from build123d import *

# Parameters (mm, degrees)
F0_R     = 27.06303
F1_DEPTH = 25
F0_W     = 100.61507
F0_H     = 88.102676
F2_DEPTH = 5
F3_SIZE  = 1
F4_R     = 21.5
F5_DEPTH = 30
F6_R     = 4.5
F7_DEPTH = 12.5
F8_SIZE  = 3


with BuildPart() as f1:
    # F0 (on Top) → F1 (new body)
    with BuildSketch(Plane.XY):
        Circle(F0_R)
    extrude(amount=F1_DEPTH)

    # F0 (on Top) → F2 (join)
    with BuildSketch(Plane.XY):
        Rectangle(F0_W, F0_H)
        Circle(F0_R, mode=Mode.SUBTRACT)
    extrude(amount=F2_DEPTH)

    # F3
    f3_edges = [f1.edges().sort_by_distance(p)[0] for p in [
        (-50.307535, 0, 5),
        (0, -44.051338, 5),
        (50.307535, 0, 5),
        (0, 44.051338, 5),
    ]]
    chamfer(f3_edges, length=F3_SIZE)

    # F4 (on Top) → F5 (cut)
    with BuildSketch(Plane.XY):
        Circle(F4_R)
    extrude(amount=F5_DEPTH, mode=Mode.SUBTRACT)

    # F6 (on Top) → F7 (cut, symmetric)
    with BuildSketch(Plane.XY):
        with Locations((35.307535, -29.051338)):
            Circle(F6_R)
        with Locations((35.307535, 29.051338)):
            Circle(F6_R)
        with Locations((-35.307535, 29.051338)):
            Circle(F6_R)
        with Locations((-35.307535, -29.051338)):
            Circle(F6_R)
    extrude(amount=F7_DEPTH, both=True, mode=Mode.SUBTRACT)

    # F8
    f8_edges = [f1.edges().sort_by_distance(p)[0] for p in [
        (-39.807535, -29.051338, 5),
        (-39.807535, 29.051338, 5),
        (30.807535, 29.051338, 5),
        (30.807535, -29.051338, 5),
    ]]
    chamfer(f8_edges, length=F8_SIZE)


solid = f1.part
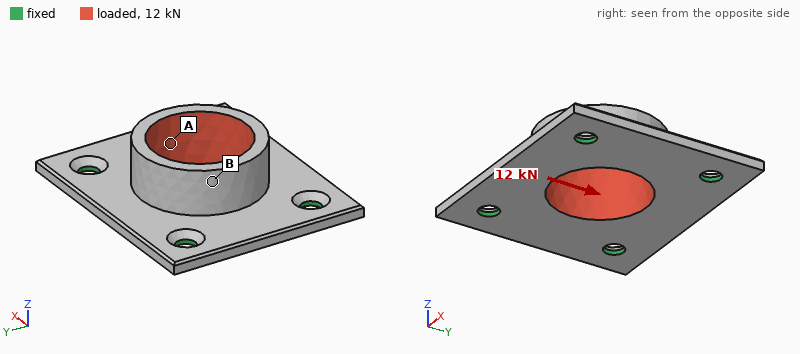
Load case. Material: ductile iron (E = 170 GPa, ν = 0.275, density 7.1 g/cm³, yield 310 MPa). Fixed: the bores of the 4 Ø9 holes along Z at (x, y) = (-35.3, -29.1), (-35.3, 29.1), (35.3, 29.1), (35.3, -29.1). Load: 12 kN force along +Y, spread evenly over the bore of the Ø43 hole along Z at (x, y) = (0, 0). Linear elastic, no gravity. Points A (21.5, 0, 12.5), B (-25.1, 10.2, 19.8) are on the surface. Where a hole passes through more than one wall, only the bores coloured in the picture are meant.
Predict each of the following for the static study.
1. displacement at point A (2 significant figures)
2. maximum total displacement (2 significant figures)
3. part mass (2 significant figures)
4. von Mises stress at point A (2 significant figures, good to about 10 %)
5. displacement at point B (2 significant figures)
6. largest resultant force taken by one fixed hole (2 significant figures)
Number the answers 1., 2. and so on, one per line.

1. 14 µm
2. 41 µm
3. 370 g
4. 31 MPa
5. 24 µm
6. 3.6 kN
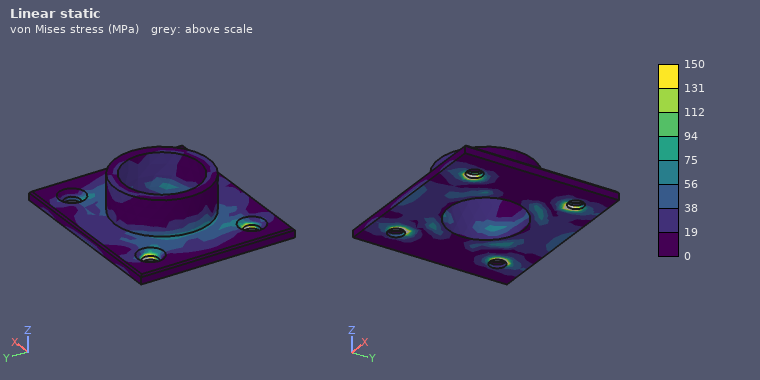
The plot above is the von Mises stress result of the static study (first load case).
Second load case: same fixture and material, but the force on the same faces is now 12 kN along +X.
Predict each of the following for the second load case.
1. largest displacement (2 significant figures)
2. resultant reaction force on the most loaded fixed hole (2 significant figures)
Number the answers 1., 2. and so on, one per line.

1. 28 µm
2. 3.4 kN
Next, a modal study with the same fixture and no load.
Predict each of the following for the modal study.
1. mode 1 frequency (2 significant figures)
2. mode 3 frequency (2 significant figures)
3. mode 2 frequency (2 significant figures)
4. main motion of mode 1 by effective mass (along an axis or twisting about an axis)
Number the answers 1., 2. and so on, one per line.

1. 4500 Hz
2. 6200 Hz
3. 4900 Hz
4. along Z
